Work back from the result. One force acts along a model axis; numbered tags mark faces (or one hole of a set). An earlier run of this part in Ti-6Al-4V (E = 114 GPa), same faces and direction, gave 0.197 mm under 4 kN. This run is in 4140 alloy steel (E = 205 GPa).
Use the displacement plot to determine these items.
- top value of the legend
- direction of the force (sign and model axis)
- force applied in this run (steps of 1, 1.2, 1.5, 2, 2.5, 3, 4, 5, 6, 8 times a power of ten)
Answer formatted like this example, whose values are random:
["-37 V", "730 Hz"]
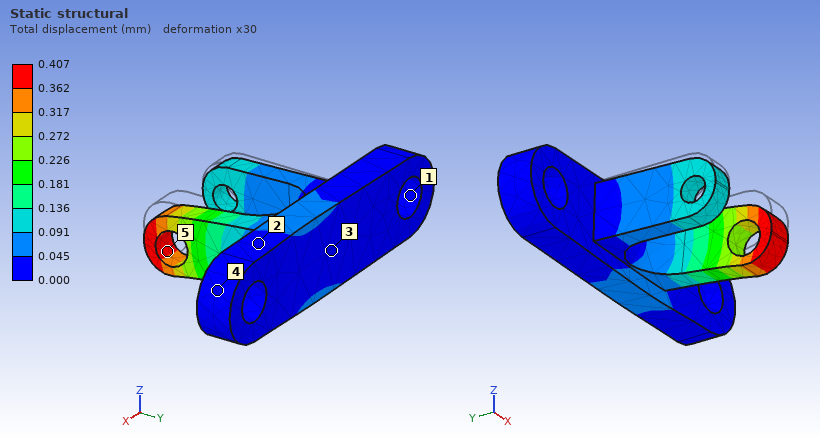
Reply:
["0.407 mm", "-Z", "15 kN"]
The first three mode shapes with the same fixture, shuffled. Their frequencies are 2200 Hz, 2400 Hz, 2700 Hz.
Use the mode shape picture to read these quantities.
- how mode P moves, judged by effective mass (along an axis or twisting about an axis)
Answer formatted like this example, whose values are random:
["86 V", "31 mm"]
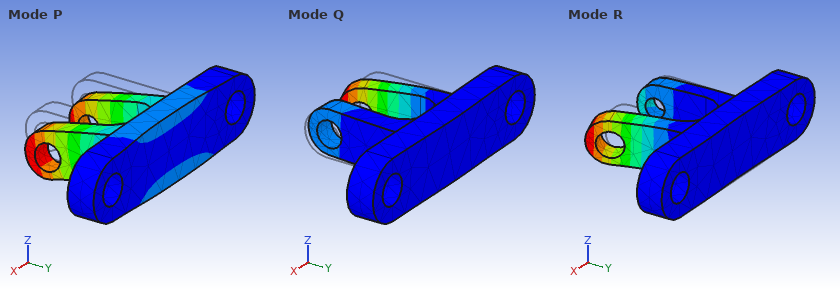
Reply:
["along Z"]
